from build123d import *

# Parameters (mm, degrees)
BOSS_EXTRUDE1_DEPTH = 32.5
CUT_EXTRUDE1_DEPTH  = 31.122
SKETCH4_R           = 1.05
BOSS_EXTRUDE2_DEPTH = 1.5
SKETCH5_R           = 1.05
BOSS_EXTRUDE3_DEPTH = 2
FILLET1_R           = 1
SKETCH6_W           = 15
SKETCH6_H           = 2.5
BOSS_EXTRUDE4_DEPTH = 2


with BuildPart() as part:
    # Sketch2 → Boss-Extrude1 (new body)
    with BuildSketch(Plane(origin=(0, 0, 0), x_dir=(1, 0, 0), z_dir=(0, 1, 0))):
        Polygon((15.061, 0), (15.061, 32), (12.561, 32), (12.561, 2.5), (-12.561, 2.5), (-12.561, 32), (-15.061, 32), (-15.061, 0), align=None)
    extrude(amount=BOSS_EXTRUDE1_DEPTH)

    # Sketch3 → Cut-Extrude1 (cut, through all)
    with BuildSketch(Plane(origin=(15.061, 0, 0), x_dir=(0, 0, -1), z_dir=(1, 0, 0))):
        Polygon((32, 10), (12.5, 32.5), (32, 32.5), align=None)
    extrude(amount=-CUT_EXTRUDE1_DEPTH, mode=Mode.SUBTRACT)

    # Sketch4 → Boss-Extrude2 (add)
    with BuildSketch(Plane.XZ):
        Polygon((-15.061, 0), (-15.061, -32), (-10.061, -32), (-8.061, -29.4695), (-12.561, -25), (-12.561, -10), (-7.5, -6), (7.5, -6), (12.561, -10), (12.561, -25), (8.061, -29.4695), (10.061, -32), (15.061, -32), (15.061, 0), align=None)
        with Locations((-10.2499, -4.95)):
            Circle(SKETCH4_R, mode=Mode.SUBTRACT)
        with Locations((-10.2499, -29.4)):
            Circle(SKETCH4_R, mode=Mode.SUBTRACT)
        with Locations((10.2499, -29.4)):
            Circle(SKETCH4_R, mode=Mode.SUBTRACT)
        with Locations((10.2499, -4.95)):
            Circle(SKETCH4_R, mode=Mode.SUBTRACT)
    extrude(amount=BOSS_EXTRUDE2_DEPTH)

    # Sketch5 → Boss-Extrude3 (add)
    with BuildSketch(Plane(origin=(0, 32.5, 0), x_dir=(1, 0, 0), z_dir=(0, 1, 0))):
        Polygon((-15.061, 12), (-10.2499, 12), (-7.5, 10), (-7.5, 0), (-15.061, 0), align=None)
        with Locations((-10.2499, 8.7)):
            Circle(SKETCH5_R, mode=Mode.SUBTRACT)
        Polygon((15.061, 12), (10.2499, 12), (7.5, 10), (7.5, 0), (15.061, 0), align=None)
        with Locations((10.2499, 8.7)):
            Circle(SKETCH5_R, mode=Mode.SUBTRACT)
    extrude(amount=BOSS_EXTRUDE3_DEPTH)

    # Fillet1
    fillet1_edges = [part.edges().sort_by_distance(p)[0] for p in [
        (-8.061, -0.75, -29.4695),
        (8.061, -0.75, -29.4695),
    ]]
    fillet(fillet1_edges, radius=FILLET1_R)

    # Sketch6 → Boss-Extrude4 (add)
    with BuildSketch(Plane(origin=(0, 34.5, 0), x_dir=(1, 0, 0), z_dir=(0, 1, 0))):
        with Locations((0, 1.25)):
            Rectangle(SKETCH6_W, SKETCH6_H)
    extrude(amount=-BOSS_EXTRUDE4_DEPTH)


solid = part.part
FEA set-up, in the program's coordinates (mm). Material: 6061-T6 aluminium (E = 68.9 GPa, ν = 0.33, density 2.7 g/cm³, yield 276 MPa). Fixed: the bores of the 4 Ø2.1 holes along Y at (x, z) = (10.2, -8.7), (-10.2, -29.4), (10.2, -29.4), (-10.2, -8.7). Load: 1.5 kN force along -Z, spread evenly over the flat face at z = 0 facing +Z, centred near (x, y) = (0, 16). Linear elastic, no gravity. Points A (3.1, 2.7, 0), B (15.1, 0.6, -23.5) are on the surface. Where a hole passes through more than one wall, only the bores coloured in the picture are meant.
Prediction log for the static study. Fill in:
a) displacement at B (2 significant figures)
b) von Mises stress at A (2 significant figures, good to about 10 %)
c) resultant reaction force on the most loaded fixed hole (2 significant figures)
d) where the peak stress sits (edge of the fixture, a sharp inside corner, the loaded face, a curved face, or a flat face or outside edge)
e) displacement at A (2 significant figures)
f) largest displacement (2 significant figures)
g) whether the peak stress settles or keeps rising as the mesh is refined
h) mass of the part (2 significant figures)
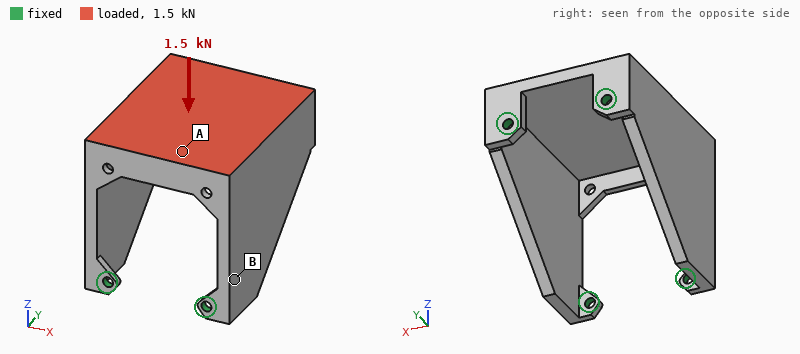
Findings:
23 µm
38 MPa
410 N
edge of the fixture
46 µm
52 µm
keeps rising
19 g
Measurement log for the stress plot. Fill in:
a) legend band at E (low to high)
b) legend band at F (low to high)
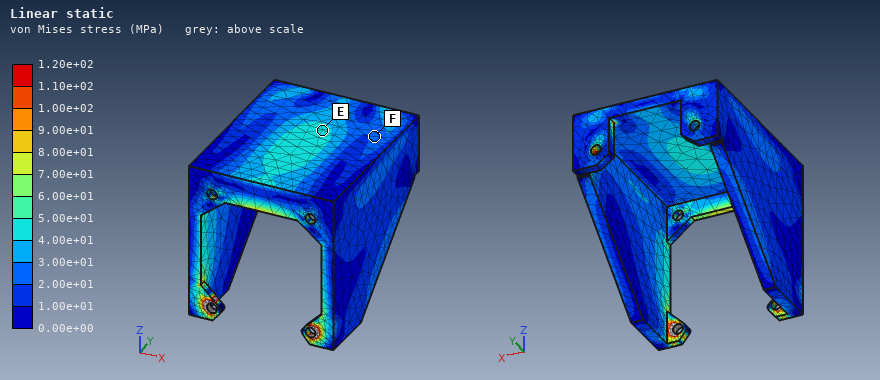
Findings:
4.00e+01 to 5.00e+01 MPa
2.00e+01 to 3.00e+01 MPa
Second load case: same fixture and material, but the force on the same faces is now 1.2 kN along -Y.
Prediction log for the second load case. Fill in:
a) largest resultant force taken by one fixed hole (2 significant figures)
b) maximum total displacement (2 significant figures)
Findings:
540 N
22 µm
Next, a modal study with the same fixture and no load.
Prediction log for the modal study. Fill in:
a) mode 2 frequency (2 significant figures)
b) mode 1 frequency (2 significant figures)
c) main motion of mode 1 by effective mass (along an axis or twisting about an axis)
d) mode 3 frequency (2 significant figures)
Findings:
7100 Hz
5400 Hz
along X
7500 Hz
